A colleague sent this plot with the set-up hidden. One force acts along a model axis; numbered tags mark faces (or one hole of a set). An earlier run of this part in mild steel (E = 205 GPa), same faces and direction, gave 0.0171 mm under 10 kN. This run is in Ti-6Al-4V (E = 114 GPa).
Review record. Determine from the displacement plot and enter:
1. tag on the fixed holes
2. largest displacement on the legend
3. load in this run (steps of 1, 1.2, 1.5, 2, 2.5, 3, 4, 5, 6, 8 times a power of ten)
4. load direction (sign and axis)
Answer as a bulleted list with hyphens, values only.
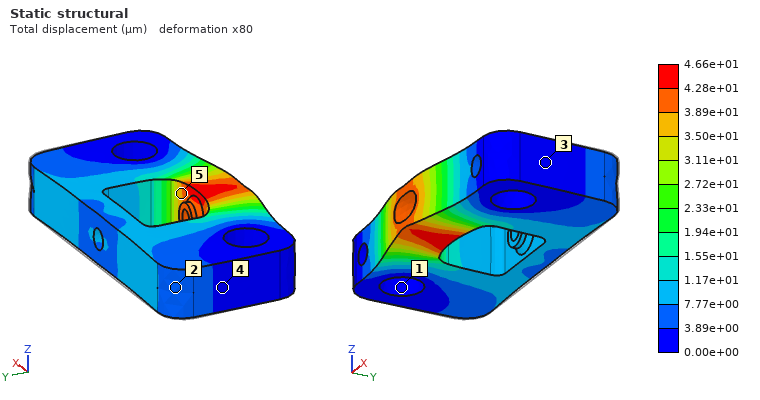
- 1
- 4.66e+01 µm
- 15 kN
- -Y
